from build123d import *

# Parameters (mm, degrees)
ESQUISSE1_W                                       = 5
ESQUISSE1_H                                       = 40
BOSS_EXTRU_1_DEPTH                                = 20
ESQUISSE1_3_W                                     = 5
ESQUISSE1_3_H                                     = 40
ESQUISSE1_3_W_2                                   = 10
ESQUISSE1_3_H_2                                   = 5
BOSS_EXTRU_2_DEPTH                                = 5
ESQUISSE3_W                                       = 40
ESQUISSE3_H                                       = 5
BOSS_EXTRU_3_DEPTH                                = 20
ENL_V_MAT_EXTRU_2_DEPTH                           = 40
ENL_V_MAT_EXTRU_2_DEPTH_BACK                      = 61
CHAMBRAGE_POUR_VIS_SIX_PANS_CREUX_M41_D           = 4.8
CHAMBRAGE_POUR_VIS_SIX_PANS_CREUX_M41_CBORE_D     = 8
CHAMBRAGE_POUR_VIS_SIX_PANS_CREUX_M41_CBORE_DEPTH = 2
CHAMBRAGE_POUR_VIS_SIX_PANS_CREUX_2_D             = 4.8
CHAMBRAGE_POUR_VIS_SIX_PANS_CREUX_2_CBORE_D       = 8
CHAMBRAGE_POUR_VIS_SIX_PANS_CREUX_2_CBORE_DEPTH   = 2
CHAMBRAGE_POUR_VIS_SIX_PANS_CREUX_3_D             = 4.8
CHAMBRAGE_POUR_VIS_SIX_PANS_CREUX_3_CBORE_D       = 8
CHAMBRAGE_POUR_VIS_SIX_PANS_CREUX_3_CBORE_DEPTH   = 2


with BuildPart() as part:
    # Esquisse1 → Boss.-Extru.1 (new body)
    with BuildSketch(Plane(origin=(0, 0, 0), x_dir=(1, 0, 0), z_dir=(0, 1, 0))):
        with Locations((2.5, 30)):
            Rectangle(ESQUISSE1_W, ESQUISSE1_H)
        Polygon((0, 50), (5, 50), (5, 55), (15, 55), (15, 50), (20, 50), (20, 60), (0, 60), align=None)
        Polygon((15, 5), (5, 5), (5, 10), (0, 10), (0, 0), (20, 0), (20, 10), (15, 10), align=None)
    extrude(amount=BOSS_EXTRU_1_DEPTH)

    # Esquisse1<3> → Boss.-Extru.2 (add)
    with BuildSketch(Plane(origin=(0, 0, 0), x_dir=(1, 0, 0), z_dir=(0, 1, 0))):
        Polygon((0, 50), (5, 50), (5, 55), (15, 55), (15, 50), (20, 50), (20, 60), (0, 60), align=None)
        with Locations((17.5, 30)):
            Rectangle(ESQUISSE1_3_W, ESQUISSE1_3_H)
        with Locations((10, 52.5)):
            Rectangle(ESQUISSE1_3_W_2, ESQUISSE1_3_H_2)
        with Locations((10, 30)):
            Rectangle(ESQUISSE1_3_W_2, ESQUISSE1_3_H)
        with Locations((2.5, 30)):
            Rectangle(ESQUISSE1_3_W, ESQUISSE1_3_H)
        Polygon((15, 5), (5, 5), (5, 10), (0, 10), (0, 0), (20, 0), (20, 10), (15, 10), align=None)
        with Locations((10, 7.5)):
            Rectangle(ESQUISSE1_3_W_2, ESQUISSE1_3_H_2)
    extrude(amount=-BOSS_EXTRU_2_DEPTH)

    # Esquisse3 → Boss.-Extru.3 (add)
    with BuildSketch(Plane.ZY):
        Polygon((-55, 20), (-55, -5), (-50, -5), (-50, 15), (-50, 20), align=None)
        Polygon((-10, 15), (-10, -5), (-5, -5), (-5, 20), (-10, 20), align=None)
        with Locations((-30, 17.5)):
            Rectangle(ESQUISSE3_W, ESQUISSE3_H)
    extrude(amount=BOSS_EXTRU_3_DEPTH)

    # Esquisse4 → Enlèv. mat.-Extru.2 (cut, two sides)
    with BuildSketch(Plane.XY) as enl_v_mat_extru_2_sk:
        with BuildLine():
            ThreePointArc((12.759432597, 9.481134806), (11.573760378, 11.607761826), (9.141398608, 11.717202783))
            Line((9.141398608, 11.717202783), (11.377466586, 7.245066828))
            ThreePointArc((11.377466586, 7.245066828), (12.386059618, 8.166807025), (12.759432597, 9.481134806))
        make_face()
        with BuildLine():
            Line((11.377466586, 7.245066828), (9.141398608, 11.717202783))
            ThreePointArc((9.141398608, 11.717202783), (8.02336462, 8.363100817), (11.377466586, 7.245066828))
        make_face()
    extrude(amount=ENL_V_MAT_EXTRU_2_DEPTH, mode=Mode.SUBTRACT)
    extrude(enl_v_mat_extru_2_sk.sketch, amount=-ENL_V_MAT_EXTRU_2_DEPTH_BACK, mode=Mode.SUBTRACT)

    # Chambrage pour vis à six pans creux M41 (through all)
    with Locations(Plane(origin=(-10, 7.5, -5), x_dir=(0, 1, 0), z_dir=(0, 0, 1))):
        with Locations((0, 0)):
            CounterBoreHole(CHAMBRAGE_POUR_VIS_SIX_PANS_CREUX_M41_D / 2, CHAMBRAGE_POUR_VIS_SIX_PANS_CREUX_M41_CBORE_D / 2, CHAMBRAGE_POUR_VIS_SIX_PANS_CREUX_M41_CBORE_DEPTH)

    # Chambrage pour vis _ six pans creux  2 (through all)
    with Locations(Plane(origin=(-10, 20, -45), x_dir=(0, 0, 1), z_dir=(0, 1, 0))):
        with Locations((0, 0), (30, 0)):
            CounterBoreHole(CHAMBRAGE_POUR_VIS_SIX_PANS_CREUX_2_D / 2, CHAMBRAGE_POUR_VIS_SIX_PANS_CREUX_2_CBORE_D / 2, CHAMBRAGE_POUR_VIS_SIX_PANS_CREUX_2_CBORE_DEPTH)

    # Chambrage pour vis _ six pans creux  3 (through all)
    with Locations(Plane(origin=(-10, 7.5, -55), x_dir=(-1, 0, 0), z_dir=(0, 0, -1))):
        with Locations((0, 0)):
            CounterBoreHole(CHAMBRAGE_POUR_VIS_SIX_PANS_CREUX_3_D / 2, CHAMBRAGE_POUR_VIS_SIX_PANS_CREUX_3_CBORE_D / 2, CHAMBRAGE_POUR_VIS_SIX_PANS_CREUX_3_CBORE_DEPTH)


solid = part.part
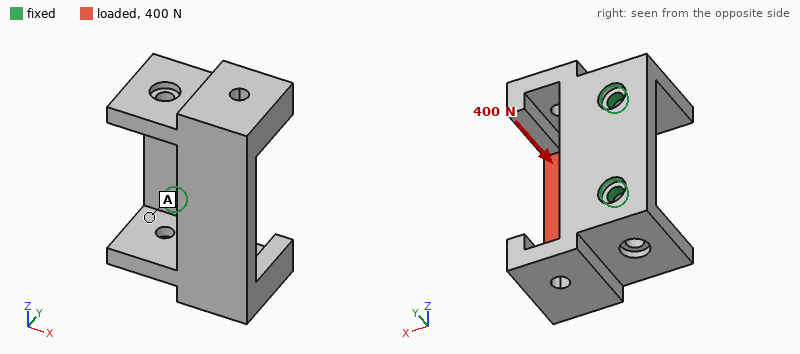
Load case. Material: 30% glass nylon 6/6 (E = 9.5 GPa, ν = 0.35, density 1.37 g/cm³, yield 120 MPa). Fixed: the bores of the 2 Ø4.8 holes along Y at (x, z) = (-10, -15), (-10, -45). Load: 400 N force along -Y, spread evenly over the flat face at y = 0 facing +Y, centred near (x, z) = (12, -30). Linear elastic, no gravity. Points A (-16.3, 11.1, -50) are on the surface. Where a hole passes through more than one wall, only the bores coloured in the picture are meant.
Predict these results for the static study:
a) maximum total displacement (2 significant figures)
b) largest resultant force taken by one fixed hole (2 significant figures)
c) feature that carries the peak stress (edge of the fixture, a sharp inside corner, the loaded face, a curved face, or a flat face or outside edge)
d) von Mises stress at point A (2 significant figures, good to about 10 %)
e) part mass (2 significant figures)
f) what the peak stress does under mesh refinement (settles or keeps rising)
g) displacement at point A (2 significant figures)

0.55 mm
210 N
edge of the fixture
10 MPa
33 g
keeps rising
0.11 mm
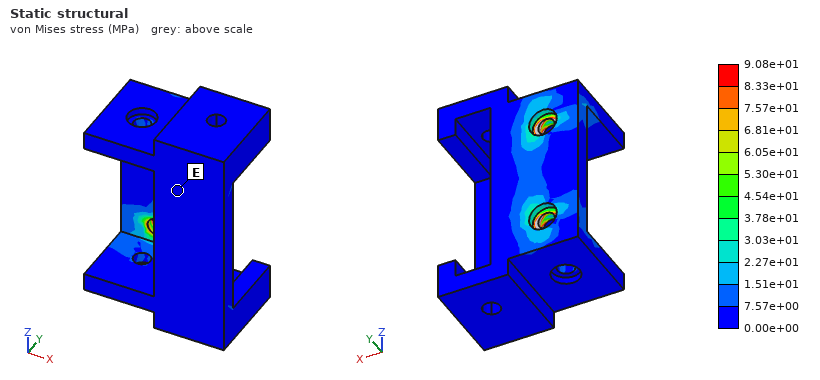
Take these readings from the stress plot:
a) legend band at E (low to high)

0.00e+00 to 7.57e+00 MPa
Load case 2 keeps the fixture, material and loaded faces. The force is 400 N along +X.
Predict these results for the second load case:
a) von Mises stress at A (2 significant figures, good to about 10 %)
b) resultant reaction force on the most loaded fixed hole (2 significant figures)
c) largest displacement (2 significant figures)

10 MPa
200 N
0.39 mm
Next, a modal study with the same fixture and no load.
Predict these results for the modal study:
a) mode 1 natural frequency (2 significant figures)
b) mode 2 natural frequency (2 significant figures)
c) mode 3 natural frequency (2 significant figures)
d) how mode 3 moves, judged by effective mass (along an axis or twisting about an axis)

1100 Hz
1800 Hz
3600 Hz
along Z
